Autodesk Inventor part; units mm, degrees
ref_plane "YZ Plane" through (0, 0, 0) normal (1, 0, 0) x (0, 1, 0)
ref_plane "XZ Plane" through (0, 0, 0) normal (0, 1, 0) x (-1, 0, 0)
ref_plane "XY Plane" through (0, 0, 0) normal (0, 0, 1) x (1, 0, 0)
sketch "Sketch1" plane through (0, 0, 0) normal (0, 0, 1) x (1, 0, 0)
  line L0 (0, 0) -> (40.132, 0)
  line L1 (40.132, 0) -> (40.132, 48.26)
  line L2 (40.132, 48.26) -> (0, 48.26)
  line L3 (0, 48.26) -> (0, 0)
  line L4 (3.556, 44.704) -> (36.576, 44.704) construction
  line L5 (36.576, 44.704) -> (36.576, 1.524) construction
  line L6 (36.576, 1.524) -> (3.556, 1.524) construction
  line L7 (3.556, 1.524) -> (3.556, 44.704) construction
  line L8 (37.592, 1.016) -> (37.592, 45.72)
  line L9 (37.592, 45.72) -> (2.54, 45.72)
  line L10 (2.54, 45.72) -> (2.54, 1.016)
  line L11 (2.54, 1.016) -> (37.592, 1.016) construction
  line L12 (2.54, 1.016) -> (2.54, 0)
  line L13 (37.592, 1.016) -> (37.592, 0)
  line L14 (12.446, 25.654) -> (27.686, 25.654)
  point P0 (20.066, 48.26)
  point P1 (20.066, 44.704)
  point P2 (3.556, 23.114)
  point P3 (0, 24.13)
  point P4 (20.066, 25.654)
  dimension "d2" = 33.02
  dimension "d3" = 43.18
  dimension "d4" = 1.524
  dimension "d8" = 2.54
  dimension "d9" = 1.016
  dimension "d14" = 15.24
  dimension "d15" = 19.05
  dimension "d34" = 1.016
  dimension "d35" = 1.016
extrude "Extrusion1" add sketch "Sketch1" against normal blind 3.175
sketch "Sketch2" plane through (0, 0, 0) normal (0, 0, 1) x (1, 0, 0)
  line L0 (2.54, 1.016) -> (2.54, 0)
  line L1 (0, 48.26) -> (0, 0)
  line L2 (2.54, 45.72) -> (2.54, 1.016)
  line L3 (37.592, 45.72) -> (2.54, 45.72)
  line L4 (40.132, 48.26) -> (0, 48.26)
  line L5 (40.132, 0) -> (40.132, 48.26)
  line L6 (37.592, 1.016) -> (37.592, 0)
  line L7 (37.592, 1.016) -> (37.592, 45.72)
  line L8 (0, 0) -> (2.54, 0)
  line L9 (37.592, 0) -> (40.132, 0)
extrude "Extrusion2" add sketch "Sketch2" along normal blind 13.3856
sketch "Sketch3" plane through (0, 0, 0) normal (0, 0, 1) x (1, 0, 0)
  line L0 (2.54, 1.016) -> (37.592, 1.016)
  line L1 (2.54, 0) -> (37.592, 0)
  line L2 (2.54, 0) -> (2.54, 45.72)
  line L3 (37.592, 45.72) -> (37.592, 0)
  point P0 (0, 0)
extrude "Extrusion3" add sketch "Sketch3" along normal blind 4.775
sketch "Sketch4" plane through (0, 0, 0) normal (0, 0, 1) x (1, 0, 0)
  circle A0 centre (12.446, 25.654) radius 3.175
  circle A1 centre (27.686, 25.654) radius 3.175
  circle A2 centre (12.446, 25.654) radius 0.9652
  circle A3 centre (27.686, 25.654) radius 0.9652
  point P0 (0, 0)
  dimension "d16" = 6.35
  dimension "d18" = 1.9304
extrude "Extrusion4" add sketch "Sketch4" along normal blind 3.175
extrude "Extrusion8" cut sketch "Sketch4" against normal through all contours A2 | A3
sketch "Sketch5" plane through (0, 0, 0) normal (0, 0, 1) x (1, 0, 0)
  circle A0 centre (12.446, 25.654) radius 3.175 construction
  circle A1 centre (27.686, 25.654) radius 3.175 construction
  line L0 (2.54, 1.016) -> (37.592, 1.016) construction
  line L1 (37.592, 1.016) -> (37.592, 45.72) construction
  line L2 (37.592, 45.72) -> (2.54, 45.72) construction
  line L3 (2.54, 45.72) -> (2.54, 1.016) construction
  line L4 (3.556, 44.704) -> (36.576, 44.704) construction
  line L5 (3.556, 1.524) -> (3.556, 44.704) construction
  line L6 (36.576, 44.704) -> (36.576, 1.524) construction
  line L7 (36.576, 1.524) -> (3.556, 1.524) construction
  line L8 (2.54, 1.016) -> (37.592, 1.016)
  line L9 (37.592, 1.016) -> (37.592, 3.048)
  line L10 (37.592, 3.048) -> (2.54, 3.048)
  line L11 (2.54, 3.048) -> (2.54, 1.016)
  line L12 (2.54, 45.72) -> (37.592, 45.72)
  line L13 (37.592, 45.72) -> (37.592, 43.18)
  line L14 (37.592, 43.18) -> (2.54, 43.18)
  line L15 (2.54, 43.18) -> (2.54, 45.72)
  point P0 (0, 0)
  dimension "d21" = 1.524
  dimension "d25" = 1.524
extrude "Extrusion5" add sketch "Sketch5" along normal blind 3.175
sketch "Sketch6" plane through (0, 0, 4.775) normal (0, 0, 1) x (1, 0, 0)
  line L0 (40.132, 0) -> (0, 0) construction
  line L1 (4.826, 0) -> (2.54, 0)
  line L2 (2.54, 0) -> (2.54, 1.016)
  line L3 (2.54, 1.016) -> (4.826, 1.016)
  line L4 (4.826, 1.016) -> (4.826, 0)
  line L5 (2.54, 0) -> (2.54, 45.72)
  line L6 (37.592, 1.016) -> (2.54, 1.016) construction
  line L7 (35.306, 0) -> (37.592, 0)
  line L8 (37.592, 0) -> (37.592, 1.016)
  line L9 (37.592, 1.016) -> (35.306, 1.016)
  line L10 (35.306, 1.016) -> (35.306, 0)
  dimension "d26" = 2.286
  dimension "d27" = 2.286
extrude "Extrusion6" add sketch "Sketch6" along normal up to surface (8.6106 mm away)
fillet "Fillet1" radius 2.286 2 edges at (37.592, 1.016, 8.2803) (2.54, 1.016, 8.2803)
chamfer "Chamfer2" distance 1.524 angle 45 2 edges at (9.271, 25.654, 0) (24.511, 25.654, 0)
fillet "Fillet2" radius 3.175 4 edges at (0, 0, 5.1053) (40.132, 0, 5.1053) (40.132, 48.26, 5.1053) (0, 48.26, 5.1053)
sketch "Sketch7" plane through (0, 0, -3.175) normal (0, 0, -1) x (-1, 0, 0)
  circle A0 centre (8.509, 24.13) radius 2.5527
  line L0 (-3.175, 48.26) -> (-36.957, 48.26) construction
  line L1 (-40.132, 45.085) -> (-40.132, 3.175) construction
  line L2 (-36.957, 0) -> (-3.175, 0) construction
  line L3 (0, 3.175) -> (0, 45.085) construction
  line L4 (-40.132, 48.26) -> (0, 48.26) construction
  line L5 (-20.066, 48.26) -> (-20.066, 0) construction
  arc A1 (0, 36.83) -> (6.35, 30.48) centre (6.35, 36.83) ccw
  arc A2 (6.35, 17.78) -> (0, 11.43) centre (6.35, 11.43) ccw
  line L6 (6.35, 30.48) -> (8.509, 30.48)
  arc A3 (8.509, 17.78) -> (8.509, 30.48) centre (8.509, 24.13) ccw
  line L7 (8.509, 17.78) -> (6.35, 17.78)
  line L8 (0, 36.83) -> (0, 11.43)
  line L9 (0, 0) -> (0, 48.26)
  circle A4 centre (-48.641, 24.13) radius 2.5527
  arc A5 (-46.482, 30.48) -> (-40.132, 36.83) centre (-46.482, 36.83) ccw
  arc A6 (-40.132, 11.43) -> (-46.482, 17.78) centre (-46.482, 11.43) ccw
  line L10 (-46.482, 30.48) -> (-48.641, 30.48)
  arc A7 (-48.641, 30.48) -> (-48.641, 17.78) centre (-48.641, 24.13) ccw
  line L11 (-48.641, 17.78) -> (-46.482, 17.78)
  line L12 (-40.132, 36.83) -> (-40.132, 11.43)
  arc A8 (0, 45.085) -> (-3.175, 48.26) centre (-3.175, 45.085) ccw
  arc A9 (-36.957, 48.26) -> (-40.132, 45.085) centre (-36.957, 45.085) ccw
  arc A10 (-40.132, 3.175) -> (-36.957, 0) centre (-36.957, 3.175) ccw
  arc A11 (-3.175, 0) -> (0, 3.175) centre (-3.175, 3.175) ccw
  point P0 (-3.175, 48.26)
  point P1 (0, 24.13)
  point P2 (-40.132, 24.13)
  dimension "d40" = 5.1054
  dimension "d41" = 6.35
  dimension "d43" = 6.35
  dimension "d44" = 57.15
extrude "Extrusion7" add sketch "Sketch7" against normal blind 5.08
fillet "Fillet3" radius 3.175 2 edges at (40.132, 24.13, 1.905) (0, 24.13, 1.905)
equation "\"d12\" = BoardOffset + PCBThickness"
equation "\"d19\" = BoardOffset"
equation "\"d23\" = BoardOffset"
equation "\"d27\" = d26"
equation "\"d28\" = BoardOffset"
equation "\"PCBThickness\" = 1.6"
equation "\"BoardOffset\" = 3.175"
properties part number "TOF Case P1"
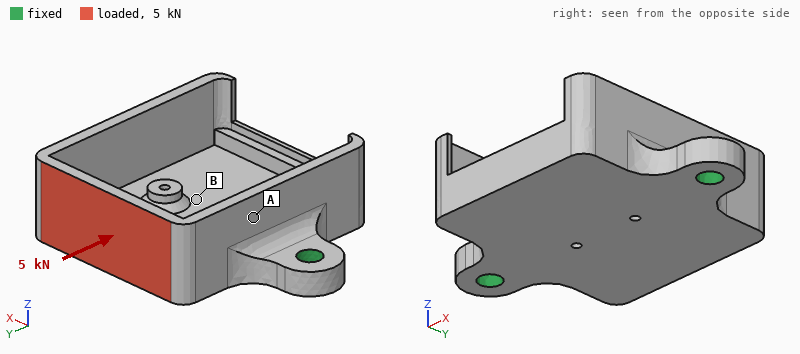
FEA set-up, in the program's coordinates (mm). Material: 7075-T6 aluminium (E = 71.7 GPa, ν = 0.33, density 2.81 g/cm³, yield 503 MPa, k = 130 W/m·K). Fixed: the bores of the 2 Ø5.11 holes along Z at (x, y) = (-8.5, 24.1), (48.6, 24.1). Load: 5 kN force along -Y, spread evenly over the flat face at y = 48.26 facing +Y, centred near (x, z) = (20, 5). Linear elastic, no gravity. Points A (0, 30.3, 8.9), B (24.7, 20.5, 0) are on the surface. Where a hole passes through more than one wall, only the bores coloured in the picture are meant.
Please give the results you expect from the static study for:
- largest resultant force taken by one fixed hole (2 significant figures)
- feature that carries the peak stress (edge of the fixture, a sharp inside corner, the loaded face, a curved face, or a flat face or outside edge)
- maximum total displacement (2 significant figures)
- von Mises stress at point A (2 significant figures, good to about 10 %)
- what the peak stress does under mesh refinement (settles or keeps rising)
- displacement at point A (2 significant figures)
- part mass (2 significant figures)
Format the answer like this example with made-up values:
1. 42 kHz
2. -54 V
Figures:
1. 2.5 kN
2. edge of the fixture
3. 0.47 mm
4. 75 MPa
5. keeps rising
6. 0.097 mm
7. 37 g
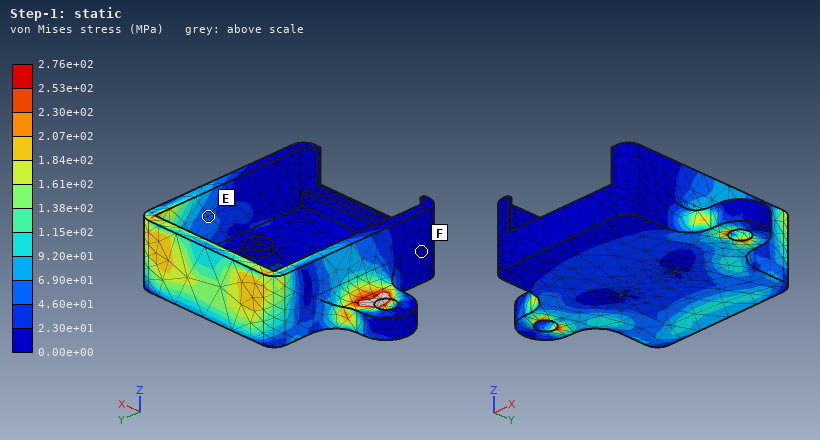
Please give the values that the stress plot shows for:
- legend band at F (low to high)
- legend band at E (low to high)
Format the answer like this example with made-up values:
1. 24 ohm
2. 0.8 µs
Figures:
1. 0.00e+00 to 2.30e+01 MPa
2. 4.60e+01 to 6.90e+01 MPa
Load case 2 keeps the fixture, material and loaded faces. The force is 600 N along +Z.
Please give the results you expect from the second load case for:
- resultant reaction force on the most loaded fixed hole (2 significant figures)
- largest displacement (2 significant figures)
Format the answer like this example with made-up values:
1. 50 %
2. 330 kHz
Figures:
1. 310 N
2. 0.13 mm
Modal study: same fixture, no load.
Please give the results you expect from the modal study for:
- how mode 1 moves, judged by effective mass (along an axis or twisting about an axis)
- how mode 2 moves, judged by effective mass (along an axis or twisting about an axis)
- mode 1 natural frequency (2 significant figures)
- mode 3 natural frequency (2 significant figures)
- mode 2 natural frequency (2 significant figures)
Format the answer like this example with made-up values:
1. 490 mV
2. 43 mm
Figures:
1. twisting about X
2. along Z
3. 3300 Hz
4. 6400 Hz
5. 5800 Hz
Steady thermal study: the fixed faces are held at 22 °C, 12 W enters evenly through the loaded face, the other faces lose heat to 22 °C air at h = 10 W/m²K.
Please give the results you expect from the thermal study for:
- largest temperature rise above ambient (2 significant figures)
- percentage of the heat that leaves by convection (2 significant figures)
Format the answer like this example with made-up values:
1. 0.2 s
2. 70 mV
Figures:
1. 19 K
2. 5.3 %
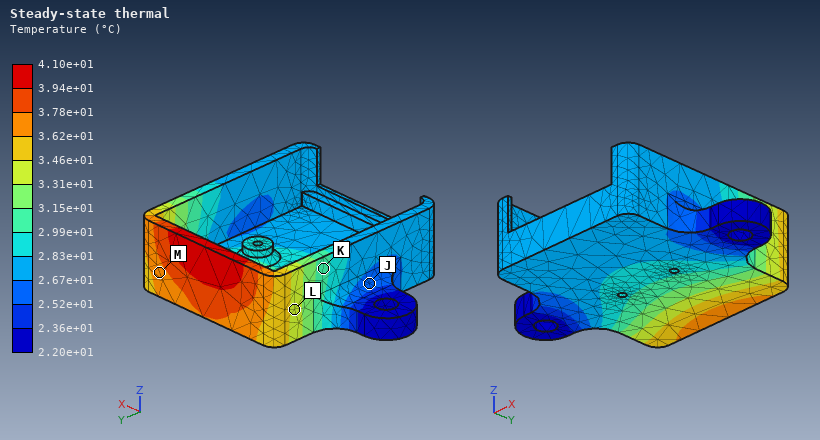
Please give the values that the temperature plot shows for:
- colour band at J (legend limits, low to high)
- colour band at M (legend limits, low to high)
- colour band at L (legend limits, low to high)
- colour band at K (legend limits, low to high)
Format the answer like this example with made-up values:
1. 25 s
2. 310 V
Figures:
1. 2.52e+01 to 2.67e+01 °C
2. 3.62e+01 to 3.78e+01 °C
3. 3.31e+01 to 3.46e+01 °C
4. 2.99e+01 to 3.15e+01 °C
